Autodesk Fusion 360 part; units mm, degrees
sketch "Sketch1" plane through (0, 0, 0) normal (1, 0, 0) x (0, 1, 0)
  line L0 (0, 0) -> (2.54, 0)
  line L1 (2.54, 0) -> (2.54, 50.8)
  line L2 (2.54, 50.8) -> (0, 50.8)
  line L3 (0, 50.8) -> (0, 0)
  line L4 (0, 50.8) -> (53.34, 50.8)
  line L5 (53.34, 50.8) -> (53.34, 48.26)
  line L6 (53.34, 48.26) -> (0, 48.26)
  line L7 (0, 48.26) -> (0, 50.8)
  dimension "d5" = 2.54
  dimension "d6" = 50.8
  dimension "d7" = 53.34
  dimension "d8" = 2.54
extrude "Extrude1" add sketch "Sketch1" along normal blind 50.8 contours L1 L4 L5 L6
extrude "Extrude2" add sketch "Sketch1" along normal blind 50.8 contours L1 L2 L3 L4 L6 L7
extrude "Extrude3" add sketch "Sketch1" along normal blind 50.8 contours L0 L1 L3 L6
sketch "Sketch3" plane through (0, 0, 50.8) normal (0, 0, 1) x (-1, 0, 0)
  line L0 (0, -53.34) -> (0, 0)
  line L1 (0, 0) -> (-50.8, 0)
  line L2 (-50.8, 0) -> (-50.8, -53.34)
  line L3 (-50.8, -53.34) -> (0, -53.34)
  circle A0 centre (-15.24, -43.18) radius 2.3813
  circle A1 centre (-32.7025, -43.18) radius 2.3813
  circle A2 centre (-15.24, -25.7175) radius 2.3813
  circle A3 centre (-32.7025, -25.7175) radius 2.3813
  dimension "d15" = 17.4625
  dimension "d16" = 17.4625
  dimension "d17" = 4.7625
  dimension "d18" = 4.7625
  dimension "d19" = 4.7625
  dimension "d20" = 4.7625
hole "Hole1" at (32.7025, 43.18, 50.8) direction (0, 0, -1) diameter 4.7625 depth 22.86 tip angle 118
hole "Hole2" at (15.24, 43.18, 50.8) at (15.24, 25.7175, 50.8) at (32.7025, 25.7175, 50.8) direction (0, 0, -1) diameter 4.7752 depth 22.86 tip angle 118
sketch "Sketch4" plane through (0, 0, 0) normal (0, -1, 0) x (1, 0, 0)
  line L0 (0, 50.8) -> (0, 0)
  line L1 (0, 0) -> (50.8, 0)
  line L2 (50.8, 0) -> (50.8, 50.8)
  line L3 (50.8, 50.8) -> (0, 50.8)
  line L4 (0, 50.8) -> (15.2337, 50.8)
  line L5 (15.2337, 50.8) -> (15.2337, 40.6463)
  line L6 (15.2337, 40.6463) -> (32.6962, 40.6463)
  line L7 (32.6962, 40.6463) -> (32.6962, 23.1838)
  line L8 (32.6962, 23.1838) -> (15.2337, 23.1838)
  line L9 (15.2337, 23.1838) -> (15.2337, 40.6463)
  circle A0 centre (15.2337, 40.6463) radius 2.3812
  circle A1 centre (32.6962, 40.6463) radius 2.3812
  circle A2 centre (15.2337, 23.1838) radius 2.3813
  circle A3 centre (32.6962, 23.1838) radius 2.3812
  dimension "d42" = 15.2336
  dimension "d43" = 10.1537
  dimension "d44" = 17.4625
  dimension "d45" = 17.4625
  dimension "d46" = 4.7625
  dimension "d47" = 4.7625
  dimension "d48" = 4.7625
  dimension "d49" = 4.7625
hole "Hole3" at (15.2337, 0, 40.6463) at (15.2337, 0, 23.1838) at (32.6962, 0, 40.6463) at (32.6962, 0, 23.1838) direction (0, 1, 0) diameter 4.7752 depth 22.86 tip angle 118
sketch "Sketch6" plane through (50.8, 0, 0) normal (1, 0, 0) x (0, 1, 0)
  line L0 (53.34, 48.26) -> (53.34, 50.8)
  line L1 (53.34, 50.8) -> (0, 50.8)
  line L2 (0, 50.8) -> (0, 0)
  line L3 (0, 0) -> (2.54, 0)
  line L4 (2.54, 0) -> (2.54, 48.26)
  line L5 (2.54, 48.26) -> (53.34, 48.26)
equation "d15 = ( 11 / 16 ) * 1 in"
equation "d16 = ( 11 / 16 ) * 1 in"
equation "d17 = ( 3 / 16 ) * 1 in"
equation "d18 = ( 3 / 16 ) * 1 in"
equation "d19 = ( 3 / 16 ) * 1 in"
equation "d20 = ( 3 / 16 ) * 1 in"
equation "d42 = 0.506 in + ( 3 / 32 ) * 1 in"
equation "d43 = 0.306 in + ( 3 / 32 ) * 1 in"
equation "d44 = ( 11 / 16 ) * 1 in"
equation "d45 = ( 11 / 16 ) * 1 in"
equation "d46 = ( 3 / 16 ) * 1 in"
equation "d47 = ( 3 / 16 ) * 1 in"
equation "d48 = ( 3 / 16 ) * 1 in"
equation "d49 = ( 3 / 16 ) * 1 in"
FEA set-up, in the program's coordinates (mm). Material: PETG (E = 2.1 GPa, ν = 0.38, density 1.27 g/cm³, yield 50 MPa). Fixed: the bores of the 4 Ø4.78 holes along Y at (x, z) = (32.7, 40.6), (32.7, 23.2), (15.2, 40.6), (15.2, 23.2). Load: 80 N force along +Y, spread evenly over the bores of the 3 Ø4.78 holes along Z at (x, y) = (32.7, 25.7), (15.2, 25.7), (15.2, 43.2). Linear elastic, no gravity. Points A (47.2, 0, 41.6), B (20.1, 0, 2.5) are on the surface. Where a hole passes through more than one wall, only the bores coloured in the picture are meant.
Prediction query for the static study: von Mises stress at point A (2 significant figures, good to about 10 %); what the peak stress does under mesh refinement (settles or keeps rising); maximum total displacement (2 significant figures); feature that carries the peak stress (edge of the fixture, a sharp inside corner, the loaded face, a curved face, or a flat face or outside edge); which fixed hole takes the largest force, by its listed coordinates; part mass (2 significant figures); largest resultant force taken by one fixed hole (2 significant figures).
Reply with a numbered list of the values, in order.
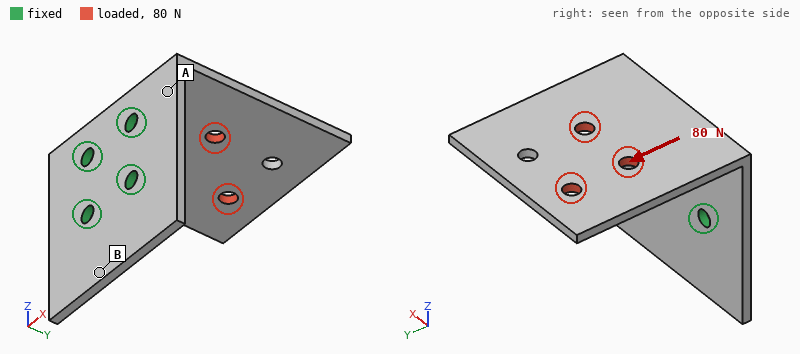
1. 2.2 MPa
2. keeps rising
3. 1.0 mm
4. edge of the fixture
5. (15.2, 40.6)
6. 16 g
7. 54 N
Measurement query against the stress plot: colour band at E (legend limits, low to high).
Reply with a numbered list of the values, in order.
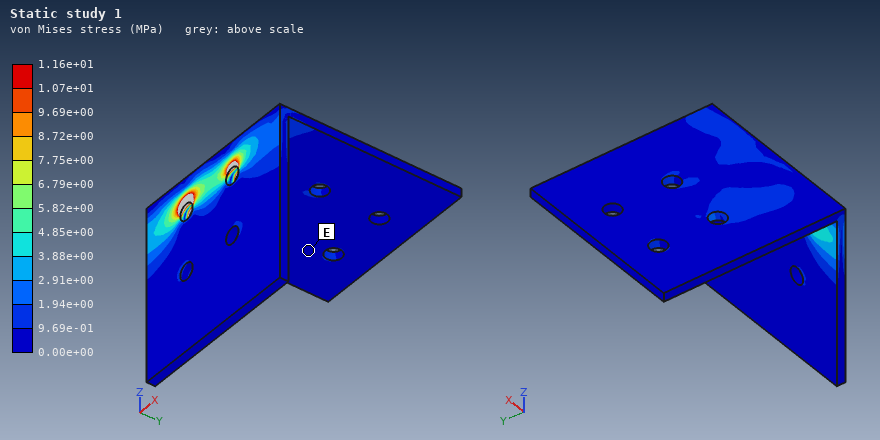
1. 0.00e+00 to 9.69e-01 MPa
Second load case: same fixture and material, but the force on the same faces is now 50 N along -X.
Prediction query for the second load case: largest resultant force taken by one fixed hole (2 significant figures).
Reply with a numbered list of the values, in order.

1. 77 N
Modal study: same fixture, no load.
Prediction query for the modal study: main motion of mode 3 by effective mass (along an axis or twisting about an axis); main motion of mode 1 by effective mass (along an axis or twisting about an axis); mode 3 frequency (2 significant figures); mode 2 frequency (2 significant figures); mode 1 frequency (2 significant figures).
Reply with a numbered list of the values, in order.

1. along X
2. along Z
3. 600 Hz
4. 410 Hz
5. 160 Hz
